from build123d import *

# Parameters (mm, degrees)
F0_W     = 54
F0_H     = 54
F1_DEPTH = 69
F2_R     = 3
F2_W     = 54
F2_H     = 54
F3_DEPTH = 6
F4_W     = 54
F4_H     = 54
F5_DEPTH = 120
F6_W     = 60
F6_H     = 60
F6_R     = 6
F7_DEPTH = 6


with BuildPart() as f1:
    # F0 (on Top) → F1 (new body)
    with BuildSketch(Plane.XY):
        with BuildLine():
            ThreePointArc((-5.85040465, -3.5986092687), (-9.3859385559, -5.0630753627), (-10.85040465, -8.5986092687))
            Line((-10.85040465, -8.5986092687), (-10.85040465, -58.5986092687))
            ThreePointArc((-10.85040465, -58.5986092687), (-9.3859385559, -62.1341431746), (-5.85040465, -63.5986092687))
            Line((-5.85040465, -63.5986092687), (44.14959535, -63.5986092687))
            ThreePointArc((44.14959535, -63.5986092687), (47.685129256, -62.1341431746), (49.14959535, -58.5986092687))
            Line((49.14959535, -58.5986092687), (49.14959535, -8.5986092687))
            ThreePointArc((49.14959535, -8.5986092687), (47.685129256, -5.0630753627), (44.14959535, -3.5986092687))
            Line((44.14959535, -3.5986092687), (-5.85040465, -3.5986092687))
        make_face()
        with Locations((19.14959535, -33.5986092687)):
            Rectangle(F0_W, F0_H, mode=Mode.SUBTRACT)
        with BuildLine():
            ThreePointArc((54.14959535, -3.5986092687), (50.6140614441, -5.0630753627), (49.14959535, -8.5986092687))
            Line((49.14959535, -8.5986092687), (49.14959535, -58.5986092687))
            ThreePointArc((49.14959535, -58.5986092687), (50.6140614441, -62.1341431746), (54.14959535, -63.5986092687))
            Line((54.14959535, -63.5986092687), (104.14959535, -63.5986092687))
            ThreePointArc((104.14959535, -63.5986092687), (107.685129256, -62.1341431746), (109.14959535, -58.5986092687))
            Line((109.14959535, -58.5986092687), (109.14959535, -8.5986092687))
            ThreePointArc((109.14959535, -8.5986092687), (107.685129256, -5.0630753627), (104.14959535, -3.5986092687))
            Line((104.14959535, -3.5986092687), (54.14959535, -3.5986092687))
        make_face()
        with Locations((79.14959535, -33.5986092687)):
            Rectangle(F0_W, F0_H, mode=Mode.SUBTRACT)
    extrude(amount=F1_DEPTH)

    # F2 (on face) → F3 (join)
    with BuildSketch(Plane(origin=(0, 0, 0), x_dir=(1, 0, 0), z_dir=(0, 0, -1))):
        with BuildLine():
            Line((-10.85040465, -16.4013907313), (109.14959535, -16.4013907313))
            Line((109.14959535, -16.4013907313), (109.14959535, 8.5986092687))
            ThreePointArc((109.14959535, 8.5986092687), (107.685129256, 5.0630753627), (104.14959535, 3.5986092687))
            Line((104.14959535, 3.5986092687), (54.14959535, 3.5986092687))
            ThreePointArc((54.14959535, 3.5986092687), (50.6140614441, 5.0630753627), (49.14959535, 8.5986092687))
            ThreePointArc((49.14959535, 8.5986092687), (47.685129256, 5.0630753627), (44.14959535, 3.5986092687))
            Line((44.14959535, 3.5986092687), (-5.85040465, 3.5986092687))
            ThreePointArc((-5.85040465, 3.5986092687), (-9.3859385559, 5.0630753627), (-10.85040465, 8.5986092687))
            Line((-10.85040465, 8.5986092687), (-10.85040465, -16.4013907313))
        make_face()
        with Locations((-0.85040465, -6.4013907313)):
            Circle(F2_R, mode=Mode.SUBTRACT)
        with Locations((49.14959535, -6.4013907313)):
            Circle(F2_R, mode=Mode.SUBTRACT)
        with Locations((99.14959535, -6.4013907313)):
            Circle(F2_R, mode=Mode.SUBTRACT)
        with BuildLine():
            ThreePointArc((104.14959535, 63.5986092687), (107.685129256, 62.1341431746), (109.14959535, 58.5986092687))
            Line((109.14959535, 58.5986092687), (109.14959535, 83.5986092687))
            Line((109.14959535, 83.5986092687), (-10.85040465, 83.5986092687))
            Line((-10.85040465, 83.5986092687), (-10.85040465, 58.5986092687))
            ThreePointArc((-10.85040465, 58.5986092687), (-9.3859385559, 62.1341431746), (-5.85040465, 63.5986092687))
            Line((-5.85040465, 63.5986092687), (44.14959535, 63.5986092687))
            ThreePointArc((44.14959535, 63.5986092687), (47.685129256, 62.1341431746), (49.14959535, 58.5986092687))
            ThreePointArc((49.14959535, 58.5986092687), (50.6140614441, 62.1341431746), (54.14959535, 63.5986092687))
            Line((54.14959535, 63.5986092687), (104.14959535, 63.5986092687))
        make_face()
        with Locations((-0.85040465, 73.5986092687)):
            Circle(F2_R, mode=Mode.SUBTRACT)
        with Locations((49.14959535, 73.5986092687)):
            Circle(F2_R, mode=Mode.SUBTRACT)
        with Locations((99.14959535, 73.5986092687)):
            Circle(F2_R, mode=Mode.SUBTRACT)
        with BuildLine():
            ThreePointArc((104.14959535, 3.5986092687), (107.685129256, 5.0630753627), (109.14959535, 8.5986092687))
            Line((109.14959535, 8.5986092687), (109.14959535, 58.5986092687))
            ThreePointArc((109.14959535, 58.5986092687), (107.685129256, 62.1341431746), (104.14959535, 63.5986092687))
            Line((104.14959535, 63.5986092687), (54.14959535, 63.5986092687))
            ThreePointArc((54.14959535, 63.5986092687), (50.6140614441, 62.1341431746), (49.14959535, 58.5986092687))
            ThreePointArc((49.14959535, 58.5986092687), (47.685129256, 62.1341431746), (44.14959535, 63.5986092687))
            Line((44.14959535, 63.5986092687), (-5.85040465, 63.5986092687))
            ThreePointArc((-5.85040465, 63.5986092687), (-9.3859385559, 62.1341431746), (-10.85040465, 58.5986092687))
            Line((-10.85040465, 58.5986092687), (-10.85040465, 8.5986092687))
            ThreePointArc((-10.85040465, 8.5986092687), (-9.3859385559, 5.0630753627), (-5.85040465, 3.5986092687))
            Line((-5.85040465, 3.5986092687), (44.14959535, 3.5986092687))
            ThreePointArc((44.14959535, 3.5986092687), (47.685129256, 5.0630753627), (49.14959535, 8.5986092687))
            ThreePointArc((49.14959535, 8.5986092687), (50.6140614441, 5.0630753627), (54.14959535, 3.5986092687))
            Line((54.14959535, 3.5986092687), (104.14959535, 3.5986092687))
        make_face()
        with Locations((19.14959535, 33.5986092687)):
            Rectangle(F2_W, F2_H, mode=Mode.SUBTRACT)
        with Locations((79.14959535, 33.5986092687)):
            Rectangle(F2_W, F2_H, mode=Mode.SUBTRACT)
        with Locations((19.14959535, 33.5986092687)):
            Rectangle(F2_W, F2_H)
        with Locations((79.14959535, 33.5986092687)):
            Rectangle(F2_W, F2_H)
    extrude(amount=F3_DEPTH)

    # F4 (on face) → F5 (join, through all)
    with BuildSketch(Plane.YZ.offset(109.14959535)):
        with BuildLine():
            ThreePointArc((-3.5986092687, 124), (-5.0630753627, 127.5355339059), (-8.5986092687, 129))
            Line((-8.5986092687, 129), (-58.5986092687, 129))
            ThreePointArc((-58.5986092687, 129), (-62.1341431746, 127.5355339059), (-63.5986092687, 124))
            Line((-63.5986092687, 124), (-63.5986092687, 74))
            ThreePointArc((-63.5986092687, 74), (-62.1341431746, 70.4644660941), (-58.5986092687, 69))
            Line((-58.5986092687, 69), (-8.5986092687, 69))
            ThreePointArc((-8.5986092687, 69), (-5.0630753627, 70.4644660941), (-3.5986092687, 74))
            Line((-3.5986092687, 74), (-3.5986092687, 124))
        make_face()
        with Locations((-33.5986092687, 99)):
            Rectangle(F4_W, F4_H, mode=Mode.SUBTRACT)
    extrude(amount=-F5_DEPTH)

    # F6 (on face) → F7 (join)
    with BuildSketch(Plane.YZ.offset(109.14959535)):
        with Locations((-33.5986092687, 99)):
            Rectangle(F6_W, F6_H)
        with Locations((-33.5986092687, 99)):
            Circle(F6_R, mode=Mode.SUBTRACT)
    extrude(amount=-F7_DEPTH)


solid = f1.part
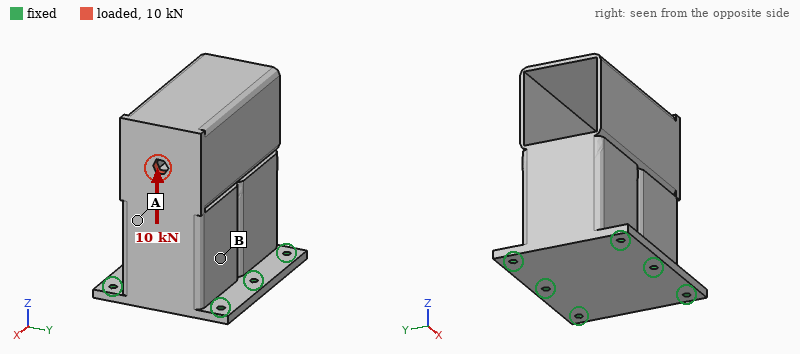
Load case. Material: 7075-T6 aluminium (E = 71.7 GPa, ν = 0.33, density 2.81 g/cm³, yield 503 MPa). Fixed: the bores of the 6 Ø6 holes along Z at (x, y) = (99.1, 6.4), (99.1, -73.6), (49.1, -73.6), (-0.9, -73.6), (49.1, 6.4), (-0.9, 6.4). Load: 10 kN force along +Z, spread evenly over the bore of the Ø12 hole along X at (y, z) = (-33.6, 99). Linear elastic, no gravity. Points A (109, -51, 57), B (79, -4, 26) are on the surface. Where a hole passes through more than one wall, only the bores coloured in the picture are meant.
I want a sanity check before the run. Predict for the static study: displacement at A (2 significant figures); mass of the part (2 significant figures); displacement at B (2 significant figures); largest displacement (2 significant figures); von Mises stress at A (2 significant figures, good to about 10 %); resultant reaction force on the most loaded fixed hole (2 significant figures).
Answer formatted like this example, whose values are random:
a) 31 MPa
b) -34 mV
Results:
a) 0.11 mm
b) 730 g
c) 0.049 mm
d) 0.18 mm
e) 40 MPa
f) 4.7 kN
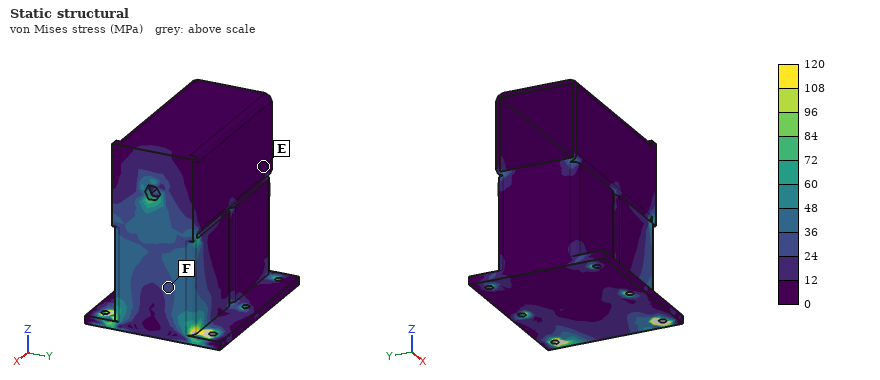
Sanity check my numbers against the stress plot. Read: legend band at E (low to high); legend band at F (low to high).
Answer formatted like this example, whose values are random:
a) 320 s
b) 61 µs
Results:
a) 0 to 12 MPa
b) 24 to 36 MPa
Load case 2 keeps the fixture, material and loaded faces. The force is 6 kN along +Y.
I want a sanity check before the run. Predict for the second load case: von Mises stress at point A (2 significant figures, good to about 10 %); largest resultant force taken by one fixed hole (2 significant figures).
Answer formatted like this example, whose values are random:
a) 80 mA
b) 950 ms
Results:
a) 37 MPa
b) 4.3 kN
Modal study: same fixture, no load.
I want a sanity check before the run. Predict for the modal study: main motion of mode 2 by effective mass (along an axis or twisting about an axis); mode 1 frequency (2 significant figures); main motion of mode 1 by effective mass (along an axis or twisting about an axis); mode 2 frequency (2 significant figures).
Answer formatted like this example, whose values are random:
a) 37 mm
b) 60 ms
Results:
a) along X
b) 1200 Hz
c) along Y
d) 1600 Hz
